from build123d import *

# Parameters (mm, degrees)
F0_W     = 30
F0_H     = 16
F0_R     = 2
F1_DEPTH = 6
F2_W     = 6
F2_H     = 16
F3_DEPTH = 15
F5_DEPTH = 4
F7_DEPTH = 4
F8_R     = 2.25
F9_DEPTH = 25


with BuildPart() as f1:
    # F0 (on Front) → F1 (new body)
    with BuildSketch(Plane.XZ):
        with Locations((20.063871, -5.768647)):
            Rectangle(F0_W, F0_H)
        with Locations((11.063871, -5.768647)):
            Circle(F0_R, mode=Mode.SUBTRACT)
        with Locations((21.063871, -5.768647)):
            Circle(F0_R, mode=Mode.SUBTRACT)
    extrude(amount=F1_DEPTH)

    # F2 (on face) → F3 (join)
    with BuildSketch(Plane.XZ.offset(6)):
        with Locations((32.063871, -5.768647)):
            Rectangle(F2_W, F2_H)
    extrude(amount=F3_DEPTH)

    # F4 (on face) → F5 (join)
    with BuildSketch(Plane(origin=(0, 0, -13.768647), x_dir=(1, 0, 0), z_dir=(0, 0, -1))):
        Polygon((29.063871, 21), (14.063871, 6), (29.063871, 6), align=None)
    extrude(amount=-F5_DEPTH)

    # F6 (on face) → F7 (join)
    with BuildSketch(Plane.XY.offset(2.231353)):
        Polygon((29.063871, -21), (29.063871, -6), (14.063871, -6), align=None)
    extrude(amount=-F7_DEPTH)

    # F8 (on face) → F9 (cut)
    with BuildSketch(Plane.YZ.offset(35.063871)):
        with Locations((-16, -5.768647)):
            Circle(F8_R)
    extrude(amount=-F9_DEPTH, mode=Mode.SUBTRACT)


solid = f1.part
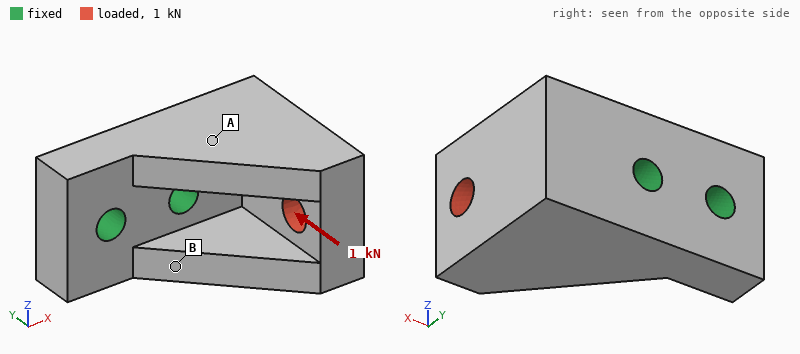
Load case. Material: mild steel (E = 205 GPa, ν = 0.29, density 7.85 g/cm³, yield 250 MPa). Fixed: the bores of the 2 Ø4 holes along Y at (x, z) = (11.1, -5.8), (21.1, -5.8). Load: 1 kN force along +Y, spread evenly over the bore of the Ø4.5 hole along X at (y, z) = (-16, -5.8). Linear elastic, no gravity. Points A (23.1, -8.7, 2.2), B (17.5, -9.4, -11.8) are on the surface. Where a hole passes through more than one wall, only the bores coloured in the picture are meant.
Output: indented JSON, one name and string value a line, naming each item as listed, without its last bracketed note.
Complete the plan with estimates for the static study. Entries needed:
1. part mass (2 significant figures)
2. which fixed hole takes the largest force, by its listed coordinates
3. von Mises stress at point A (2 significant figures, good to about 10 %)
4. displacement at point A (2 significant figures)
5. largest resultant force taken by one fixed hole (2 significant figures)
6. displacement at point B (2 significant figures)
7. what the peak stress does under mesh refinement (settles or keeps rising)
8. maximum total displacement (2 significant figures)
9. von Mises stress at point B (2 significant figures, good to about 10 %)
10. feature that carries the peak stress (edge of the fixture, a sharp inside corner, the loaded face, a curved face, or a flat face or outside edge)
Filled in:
{
  "part mass": "39 g",
  "which fixed hole takes the largest force, by its listed coordinates": "(21.1, -5.8)",
  "von Mises stress at point A": "14 MPa",
  "displacement at point A": "2.3 µm",
  "largest resultant force taken by one fixed hole": "1.4 kN",
  "displacement at point B": "1.8 µm",
  "what the peak stress does under mesh refinement": "keeps rising",
  "maximum total displacement": "11 µm",
  "von Mises stress at point B": "30 MPa",
  "feature that carries the peak stress": "edge of the fixture"
}
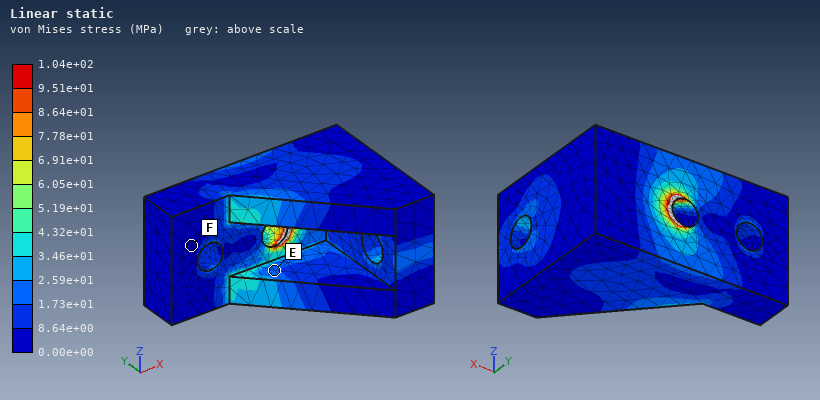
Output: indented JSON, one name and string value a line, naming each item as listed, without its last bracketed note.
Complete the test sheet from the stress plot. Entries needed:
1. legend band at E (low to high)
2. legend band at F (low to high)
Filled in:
{
  "legend band at E": "1.73e+01 to 2.59e+01 MPa",
  "legend band at F": "0.00e+00 to 8.64e+00 MPa"
}
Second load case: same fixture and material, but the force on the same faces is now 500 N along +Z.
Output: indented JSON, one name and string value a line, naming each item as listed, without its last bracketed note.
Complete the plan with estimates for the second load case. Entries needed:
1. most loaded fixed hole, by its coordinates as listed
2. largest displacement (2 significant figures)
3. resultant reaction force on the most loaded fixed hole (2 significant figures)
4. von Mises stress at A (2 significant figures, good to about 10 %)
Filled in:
{
  "most loaded fixed hole, by its coordinates as listed": "(21.1, -5.8)",
  "largest displacement": "10 µm",
  "resultant reaction force on the most loaded fixed hole": "810 N",
  "von Mises stress at A": "20 MPa"
}
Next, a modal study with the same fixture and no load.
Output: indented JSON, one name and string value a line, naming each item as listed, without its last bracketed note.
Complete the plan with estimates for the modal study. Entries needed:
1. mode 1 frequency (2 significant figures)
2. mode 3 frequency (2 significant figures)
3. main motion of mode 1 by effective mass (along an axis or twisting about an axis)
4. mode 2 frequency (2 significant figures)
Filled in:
{
  "mode 1 frequency": "12 kHz",
  "mode 3 frequency": "23 kHz",
  "main motion of mode 1 by effective mass": "along Z",
  "mode 2 frequency": "13 kHz"
}
